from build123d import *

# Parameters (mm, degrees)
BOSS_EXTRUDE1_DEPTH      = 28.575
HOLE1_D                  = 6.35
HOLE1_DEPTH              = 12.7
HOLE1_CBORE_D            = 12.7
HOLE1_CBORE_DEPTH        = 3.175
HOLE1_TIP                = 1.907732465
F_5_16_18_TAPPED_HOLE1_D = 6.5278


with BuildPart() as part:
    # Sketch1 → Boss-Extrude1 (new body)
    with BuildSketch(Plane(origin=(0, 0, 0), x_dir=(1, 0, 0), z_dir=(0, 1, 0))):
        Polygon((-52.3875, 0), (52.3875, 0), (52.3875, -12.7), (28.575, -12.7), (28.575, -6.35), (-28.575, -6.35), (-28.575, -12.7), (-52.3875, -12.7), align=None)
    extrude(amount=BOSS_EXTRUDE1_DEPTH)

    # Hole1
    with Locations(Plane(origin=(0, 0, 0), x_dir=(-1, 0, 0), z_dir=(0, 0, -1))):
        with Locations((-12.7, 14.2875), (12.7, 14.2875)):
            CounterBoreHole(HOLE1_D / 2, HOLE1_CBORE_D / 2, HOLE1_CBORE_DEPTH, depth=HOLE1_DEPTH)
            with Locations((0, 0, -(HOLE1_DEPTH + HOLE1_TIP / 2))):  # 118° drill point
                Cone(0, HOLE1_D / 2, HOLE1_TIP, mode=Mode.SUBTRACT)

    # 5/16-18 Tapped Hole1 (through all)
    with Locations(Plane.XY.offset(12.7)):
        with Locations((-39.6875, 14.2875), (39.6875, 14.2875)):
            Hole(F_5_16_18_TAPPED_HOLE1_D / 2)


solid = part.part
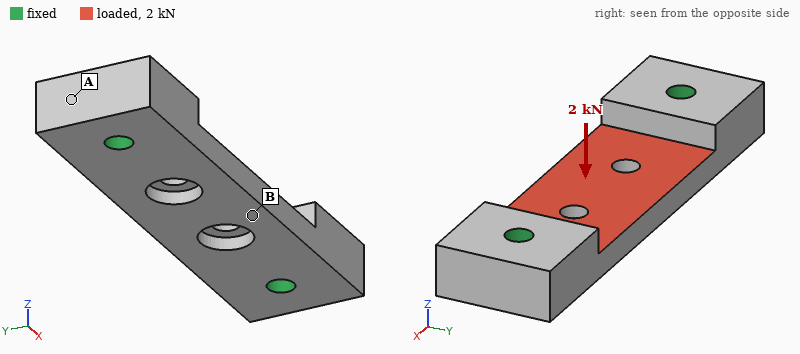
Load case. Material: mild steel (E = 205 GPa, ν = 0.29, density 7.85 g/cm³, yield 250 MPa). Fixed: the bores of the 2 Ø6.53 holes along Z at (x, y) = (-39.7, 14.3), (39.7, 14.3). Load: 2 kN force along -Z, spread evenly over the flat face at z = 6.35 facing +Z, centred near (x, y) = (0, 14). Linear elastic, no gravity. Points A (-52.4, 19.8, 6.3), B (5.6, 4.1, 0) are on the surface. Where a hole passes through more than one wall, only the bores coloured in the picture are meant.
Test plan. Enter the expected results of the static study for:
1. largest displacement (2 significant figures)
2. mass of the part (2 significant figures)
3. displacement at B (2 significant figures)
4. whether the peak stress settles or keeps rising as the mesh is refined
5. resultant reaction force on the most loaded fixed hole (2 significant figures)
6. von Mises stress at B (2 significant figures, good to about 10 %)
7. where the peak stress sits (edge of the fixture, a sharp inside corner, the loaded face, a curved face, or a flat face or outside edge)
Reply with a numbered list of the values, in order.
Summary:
1. 17 µm
2. 200 g
3. 15 µm
4. keeps rising
5. 1.0 kN
6. 36 MPa
7. edge of the fixture
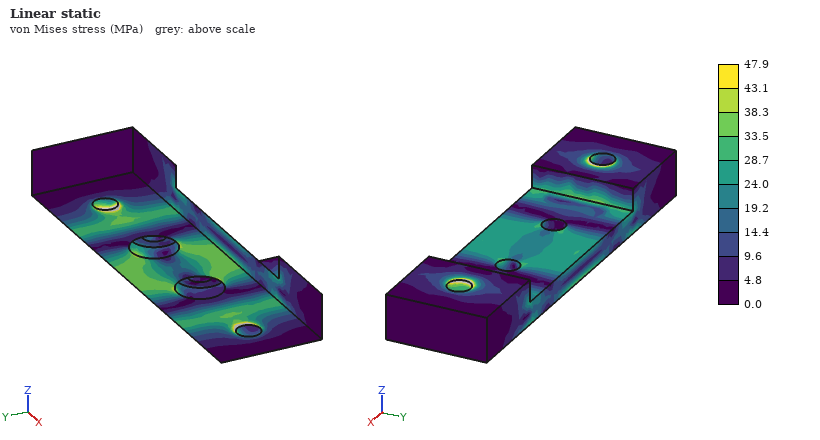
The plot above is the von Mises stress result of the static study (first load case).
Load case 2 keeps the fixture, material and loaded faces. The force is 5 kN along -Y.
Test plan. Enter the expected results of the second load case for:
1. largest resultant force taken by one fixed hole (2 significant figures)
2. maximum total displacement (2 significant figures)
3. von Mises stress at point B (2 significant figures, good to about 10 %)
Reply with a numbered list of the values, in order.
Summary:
1. 2.5 kN
2. 16 µm
3. 36 MPa
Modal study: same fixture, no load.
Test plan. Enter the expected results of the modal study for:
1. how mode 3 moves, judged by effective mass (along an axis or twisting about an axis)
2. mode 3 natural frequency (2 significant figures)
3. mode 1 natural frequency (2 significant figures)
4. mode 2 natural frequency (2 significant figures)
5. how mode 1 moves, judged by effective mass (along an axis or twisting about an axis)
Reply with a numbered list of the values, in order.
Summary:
1. along Y
2. 13 kHz
3. 7300 Hz
4. 11 kHz
5. along Z
